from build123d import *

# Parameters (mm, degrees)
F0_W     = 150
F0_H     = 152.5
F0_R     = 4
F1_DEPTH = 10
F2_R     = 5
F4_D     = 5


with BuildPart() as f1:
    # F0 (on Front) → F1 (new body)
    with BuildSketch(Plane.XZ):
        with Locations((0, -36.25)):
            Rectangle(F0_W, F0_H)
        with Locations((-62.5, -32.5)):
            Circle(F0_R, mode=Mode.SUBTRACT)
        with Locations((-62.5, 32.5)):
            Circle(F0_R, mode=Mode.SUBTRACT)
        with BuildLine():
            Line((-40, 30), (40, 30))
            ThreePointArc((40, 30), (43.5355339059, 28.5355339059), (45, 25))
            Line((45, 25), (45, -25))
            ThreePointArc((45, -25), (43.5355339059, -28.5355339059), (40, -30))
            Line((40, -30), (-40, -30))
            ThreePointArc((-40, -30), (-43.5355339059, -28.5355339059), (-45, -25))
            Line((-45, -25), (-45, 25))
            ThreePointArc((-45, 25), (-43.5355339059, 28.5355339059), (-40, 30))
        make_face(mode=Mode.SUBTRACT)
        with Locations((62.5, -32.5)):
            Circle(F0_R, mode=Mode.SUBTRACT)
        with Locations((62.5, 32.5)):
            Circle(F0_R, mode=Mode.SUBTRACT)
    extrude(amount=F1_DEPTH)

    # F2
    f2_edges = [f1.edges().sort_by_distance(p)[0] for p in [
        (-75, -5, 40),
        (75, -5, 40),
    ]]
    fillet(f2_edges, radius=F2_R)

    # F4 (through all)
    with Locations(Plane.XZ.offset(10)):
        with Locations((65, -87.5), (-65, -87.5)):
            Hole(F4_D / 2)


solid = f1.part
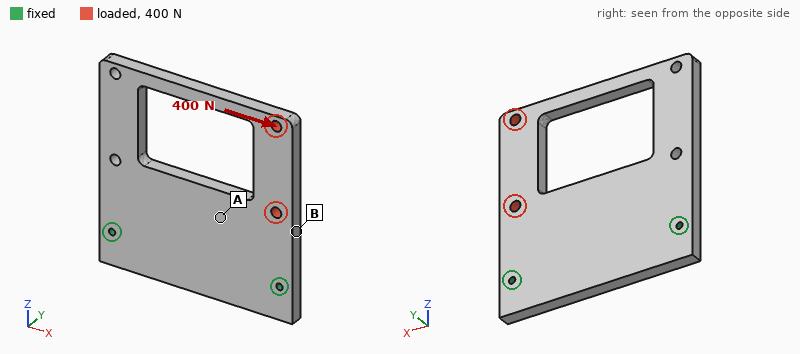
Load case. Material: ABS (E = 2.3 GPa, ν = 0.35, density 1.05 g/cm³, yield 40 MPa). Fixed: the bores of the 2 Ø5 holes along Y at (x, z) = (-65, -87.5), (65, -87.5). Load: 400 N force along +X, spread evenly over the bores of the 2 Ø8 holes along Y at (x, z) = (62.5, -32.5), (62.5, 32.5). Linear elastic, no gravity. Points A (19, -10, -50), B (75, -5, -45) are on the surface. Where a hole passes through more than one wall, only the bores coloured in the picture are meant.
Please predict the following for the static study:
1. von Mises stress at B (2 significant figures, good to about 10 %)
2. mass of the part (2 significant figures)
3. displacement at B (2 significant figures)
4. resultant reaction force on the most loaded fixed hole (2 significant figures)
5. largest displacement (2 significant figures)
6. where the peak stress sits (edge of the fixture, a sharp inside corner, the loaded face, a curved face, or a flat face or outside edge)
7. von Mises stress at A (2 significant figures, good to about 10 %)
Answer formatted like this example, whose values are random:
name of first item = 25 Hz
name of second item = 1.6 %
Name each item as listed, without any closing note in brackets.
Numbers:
von Mises stress at B = 3.2 MPa
mass of the part = 180 g
displacement at B = 0.065 mm
resultant reaction force on the most loaded fixed hole = 340 N
largest displacement = 0.43 mm
where the peak stress sits = a curved face
von Mises stress at A = 1.1 MPa
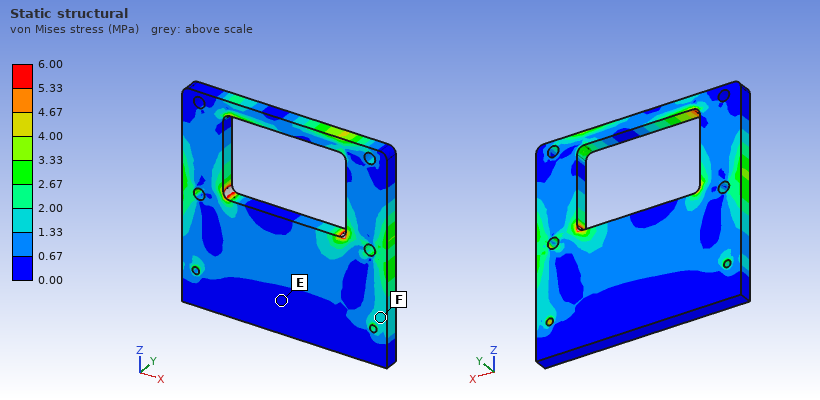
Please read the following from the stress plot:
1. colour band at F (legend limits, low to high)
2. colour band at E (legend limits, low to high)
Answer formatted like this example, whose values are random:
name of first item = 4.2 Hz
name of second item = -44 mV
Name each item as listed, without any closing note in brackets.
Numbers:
colour band at F = 1.33 to 2.00 MPa
colour band at E = 0.00 to 0.67 MPa
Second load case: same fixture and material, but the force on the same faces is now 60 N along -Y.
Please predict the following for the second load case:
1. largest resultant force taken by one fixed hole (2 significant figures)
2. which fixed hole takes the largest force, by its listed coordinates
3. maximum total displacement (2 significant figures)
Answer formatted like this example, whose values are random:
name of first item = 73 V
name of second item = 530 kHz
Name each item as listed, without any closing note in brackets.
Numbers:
largest resultant force taken by one fixed hole = 60 N
which fixed hole takes the largest force, by its listed coordinates = (65, -87.5)
maximum total displacement = 2.4 mm
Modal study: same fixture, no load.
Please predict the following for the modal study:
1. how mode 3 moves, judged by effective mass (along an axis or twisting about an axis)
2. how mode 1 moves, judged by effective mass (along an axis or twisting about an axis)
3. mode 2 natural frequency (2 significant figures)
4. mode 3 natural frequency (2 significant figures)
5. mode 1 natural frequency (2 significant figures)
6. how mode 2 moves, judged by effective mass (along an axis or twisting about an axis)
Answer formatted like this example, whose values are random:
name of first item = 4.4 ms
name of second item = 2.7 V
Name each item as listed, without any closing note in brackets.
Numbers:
how mode 3 moves, judged by effective mass = along Y
how mode 1 moves, judged by effective mass = along Y
mode 2 natural frequency = 260 Hz
mode 3 natural frequency = 560 Hz
mode 1 natural frequency = 140 Hz
how mode 2 moves, judged by effective mass = twisting about Z
